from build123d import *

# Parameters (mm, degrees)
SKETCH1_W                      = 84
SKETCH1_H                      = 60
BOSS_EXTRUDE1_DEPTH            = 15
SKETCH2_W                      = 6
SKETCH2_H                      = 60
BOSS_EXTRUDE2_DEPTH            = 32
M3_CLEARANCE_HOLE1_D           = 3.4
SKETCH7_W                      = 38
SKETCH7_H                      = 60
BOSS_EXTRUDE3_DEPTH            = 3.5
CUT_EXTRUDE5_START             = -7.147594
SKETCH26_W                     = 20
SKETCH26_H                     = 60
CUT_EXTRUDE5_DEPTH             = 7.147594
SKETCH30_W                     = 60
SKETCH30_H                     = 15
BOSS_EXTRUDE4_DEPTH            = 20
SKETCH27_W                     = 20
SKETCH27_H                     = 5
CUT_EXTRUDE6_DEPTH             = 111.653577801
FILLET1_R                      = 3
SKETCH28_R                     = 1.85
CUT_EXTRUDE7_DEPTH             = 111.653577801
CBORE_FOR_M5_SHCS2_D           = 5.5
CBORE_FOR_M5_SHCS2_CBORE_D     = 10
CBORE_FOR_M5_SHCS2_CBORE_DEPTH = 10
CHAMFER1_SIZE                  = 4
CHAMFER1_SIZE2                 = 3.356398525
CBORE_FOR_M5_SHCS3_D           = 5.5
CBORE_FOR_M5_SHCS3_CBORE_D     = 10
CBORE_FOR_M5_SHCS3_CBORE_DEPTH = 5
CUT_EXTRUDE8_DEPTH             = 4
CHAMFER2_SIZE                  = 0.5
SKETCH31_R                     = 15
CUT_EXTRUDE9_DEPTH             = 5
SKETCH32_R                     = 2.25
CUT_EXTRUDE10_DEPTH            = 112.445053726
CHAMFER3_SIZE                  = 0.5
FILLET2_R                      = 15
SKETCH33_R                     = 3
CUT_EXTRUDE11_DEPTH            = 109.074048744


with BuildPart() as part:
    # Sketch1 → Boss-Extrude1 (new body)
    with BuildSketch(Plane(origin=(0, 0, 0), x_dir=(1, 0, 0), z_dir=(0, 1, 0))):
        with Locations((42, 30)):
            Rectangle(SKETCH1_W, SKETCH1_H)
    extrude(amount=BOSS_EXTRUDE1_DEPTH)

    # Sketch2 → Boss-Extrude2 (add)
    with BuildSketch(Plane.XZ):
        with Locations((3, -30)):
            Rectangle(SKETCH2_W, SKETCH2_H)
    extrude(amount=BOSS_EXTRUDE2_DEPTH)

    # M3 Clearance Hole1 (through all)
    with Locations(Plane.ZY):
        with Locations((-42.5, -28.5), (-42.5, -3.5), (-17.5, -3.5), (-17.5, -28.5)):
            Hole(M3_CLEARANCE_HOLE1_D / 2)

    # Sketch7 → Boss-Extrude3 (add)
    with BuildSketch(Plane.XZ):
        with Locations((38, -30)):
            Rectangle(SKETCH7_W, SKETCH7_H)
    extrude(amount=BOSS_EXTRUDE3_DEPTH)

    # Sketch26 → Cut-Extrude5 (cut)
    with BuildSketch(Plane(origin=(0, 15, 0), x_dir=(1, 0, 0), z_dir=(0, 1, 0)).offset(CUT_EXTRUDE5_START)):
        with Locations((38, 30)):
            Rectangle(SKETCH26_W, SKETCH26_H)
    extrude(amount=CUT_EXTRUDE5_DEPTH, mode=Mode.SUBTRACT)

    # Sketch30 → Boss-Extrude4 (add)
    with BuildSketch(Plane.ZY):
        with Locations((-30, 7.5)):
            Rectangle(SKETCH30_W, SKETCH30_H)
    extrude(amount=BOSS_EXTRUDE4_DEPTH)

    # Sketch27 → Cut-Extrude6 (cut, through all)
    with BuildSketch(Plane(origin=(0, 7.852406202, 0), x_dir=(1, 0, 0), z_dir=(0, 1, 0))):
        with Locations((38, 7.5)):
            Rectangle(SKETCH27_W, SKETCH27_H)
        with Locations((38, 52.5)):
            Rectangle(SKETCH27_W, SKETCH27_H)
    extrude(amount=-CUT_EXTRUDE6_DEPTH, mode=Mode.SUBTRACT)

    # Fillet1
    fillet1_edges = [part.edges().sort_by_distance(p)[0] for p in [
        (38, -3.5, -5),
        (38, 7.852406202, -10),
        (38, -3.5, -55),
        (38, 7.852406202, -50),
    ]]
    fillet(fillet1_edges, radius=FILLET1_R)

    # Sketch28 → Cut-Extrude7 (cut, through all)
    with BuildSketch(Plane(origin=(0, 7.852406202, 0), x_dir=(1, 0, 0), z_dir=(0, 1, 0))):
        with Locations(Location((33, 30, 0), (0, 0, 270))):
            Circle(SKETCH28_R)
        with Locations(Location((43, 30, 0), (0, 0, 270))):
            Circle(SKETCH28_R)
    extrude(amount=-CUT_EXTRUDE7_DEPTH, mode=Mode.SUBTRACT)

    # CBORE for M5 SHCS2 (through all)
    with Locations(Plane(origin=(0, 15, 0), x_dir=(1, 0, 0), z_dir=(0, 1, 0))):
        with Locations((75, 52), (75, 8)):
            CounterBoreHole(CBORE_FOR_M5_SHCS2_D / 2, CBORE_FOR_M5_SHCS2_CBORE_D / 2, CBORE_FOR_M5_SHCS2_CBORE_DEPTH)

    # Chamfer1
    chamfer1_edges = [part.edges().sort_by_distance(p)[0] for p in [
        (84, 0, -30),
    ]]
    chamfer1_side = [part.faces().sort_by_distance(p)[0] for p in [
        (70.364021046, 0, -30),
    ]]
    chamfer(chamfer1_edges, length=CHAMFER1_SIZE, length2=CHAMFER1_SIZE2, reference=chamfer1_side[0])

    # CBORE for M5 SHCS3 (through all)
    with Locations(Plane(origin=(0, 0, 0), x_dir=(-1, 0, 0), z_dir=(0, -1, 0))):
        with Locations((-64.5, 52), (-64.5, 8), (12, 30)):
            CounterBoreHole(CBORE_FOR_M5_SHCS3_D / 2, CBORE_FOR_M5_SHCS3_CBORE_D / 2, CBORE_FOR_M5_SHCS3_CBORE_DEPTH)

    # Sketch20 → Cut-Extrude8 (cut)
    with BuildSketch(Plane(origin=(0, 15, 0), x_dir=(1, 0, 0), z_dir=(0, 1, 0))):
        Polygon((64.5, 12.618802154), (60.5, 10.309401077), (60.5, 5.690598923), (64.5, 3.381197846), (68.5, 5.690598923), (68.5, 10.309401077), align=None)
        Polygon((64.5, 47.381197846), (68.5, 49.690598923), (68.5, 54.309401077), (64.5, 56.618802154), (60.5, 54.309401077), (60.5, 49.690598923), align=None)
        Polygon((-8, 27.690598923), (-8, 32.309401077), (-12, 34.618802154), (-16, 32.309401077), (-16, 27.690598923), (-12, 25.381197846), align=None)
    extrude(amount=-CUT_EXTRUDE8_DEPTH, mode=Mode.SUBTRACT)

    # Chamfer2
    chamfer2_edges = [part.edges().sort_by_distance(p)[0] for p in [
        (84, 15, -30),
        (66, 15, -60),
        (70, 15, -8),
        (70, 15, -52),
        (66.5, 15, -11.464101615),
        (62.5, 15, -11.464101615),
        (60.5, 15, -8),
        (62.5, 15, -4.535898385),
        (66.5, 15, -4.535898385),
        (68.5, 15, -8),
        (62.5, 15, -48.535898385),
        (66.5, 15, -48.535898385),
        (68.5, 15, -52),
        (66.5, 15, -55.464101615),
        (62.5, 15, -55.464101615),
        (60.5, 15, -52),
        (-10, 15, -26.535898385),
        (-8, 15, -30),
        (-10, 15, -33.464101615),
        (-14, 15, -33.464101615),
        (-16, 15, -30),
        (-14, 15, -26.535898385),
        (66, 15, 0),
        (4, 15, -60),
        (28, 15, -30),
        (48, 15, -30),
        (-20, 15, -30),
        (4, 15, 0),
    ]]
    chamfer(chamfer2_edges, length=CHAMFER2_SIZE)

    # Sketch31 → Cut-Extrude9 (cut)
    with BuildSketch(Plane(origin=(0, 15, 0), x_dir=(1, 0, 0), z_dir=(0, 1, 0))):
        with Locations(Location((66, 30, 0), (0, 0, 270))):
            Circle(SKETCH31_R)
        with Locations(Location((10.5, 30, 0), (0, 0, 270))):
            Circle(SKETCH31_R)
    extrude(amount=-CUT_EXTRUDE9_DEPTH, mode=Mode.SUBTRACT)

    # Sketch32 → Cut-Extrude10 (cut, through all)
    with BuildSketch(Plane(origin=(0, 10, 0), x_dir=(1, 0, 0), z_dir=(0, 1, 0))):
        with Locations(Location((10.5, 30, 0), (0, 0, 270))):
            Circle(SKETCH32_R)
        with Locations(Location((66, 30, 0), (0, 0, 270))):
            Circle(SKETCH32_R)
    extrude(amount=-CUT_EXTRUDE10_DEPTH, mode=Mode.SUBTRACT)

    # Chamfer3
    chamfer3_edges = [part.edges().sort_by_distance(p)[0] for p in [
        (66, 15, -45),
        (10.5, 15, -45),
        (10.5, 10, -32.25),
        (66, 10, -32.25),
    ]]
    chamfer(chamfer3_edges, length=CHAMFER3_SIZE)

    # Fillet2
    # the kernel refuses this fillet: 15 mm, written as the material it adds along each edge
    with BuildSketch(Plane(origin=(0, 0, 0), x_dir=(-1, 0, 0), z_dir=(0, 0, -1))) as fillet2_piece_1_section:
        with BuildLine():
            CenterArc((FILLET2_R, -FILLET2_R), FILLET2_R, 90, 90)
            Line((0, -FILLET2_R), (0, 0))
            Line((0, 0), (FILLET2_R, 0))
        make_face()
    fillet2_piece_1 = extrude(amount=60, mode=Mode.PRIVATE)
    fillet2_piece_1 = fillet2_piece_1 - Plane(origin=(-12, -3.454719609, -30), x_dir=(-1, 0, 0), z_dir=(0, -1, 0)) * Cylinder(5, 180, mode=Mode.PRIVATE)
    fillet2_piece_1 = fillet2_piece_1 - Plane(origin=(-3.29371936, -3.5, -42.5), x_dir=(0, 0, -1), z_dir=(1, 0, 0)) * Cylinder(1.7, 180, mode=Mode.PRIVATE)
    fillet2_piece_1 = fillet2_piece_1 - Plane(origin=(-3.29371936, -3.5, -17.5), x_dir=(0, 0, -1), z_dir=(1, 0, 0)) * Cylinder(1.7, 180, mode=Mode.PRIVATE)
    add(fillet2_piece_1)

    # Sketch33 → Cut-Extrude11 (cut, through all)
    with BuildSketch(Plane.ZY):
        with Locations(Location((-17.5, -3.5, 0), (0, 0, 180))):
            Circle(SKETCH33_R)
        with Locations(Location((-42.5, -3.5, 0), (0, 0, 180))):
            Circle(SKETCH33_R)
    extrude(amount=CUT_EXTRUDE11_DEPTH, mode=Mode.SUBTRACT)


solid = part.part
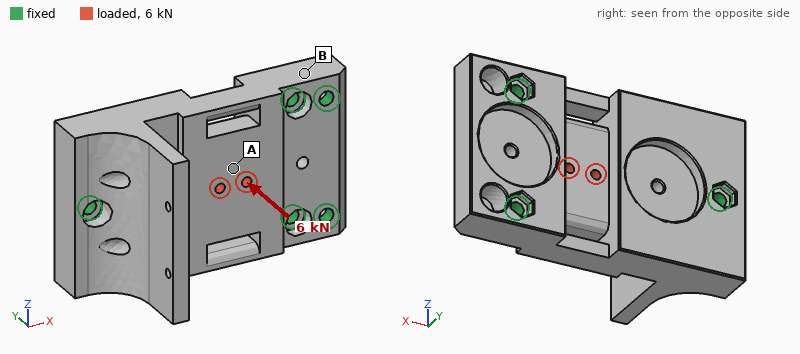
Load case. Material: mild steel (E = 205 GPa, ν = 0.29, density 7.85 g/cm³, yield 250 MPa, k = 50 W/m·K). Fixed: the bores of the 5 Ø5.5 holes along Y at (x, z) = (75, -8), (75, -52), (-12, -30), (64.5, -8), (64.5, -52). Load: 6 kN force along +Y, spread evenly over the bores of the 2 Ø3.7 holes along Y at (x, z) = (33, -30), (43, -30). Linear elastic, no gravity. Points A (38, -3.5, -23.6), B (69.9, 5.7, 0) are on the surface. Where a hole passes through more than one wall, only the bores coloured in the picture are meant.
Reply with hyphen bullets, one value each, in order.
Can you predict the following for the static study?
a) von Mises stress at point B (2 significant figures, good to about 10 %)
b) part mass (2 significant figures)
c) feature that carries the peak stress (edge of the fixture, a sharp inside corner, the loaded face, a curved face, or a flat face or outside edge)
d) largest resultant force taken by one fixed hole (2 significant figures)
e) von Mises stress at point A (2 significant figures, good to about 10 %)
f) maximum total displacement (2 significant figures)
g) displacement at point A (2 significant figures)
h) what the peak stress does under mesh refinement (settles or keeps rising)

- 16 MPa
- 720 g
- edge of the fixture
- 3.8 kN
- 44 MPa
- 17 µm
- 15 µm
- keeps rising
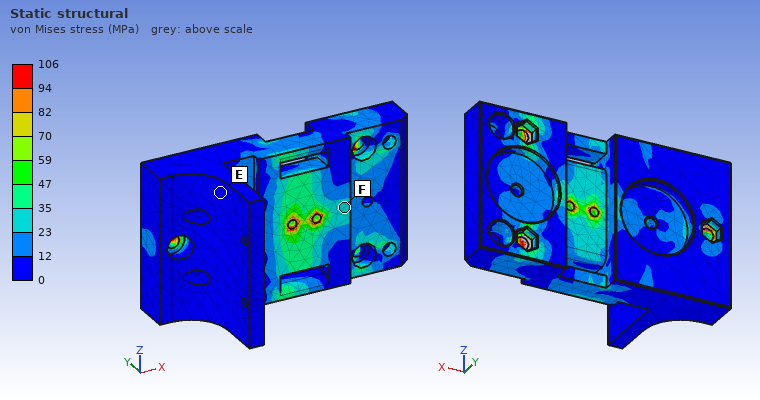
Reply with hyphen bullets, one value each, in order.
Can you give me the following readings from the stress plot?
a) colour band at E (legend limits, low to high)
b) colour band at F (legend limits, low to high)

- 0 to 12 MPa
- 23 to 35 MPa
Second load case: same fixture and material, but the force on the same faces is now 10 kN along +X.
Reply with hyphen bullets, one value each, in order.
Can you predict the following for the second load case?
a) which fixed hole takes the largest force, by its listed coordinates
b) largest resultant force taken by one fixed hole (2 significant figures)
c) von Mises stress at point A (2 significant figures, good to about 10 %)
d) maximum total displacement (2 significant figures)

- (-12, -30)
- 3.6 kN
- 19 MPa
- 5.0 µm
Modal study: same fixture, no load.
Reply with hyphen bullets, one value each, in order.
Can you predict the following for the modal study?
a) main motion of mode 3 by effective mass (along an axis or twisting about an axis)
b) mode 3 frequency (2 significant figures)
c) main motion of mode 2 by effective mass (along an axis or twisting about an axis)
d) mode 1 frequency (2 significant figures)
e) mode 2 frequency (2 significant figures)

- along Y
- 7500 Hz
- along Y
- 3600 Hz
- 4900 Hz
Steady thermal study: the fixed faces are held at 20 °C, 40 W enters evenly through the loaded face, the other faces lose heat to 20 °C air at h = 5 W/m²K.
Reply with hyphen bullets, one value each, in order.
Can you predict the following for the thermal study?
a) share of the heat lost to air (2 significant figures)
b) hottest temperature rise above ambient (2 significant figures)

- 3.7 %
- 38 K
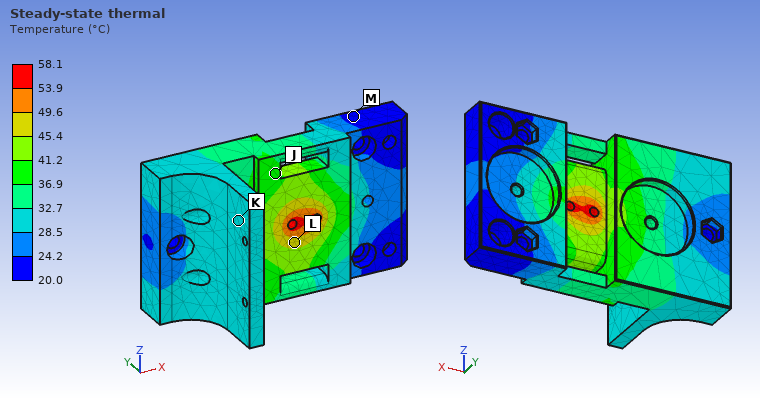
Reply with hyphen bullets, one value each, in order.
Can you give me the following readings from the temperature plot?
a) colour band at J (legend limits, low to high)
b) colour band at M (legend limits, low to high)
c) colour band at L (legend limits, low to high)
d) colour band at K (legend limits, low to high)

- 36.9 to 41.2 °C
- 20.0 to 24.2 °C
- 45.4 to 49.6 °C
- 28.5 to 32.7 °C
